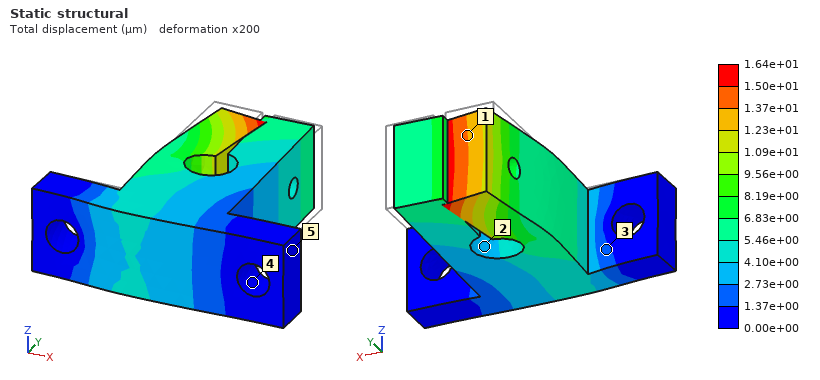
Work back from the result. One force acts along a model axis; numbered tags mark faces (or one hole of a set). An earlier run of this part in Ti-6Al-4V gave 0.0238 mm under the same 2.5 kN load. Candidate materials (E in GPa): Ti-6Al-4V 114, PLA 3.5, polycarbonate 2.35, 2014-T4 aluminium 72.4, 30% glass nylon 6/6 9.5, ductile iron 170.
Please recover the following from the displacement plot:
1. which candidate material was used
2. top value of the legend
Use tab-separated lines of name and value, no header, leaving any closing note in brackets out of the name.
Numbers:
which candidate material was used	ductile iron
top value of the legend	1.64e+01 µm
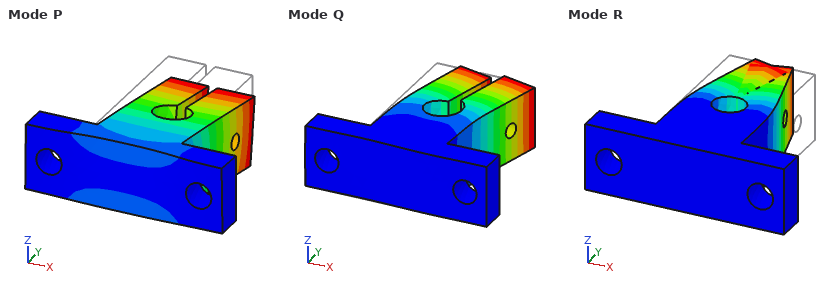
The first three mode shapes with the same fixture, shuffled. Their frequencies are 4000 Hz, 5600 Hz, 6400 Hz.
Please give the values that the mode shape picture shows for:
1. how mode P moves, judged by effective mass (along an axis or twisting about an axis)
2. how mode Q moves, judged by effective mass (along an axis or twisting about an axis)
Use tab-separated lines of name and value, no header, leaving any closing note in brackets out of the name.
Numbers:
how mode P moves, judged by effective mass	along Z
how mode Q moves, judged by effective mass	along X
